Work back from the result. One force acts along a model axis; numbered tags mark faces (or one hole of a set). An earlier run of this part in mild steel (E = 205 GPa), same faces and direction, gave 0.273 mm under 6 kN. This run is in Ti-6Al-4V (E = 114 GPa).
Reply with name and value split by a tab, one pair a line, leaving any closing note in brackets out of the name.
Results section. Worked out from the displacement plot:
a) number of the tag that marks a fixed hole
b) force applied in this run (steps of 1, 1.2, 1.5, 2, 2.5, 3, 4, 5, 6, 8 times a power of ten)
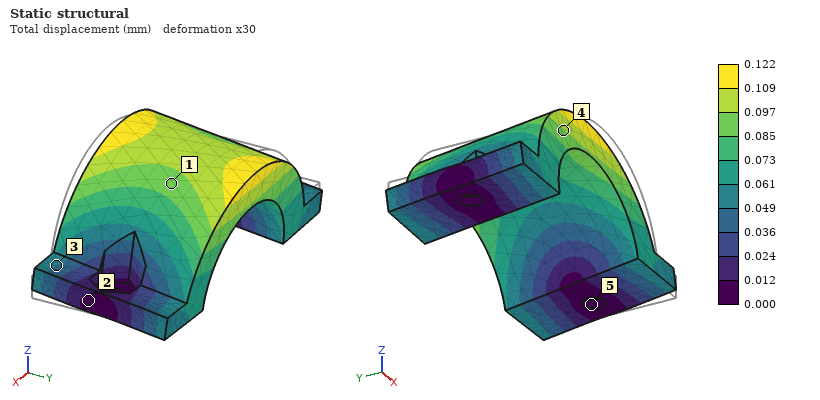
number of the tag that marks a fixed hole	5
force applied in this run	1.5 kN
